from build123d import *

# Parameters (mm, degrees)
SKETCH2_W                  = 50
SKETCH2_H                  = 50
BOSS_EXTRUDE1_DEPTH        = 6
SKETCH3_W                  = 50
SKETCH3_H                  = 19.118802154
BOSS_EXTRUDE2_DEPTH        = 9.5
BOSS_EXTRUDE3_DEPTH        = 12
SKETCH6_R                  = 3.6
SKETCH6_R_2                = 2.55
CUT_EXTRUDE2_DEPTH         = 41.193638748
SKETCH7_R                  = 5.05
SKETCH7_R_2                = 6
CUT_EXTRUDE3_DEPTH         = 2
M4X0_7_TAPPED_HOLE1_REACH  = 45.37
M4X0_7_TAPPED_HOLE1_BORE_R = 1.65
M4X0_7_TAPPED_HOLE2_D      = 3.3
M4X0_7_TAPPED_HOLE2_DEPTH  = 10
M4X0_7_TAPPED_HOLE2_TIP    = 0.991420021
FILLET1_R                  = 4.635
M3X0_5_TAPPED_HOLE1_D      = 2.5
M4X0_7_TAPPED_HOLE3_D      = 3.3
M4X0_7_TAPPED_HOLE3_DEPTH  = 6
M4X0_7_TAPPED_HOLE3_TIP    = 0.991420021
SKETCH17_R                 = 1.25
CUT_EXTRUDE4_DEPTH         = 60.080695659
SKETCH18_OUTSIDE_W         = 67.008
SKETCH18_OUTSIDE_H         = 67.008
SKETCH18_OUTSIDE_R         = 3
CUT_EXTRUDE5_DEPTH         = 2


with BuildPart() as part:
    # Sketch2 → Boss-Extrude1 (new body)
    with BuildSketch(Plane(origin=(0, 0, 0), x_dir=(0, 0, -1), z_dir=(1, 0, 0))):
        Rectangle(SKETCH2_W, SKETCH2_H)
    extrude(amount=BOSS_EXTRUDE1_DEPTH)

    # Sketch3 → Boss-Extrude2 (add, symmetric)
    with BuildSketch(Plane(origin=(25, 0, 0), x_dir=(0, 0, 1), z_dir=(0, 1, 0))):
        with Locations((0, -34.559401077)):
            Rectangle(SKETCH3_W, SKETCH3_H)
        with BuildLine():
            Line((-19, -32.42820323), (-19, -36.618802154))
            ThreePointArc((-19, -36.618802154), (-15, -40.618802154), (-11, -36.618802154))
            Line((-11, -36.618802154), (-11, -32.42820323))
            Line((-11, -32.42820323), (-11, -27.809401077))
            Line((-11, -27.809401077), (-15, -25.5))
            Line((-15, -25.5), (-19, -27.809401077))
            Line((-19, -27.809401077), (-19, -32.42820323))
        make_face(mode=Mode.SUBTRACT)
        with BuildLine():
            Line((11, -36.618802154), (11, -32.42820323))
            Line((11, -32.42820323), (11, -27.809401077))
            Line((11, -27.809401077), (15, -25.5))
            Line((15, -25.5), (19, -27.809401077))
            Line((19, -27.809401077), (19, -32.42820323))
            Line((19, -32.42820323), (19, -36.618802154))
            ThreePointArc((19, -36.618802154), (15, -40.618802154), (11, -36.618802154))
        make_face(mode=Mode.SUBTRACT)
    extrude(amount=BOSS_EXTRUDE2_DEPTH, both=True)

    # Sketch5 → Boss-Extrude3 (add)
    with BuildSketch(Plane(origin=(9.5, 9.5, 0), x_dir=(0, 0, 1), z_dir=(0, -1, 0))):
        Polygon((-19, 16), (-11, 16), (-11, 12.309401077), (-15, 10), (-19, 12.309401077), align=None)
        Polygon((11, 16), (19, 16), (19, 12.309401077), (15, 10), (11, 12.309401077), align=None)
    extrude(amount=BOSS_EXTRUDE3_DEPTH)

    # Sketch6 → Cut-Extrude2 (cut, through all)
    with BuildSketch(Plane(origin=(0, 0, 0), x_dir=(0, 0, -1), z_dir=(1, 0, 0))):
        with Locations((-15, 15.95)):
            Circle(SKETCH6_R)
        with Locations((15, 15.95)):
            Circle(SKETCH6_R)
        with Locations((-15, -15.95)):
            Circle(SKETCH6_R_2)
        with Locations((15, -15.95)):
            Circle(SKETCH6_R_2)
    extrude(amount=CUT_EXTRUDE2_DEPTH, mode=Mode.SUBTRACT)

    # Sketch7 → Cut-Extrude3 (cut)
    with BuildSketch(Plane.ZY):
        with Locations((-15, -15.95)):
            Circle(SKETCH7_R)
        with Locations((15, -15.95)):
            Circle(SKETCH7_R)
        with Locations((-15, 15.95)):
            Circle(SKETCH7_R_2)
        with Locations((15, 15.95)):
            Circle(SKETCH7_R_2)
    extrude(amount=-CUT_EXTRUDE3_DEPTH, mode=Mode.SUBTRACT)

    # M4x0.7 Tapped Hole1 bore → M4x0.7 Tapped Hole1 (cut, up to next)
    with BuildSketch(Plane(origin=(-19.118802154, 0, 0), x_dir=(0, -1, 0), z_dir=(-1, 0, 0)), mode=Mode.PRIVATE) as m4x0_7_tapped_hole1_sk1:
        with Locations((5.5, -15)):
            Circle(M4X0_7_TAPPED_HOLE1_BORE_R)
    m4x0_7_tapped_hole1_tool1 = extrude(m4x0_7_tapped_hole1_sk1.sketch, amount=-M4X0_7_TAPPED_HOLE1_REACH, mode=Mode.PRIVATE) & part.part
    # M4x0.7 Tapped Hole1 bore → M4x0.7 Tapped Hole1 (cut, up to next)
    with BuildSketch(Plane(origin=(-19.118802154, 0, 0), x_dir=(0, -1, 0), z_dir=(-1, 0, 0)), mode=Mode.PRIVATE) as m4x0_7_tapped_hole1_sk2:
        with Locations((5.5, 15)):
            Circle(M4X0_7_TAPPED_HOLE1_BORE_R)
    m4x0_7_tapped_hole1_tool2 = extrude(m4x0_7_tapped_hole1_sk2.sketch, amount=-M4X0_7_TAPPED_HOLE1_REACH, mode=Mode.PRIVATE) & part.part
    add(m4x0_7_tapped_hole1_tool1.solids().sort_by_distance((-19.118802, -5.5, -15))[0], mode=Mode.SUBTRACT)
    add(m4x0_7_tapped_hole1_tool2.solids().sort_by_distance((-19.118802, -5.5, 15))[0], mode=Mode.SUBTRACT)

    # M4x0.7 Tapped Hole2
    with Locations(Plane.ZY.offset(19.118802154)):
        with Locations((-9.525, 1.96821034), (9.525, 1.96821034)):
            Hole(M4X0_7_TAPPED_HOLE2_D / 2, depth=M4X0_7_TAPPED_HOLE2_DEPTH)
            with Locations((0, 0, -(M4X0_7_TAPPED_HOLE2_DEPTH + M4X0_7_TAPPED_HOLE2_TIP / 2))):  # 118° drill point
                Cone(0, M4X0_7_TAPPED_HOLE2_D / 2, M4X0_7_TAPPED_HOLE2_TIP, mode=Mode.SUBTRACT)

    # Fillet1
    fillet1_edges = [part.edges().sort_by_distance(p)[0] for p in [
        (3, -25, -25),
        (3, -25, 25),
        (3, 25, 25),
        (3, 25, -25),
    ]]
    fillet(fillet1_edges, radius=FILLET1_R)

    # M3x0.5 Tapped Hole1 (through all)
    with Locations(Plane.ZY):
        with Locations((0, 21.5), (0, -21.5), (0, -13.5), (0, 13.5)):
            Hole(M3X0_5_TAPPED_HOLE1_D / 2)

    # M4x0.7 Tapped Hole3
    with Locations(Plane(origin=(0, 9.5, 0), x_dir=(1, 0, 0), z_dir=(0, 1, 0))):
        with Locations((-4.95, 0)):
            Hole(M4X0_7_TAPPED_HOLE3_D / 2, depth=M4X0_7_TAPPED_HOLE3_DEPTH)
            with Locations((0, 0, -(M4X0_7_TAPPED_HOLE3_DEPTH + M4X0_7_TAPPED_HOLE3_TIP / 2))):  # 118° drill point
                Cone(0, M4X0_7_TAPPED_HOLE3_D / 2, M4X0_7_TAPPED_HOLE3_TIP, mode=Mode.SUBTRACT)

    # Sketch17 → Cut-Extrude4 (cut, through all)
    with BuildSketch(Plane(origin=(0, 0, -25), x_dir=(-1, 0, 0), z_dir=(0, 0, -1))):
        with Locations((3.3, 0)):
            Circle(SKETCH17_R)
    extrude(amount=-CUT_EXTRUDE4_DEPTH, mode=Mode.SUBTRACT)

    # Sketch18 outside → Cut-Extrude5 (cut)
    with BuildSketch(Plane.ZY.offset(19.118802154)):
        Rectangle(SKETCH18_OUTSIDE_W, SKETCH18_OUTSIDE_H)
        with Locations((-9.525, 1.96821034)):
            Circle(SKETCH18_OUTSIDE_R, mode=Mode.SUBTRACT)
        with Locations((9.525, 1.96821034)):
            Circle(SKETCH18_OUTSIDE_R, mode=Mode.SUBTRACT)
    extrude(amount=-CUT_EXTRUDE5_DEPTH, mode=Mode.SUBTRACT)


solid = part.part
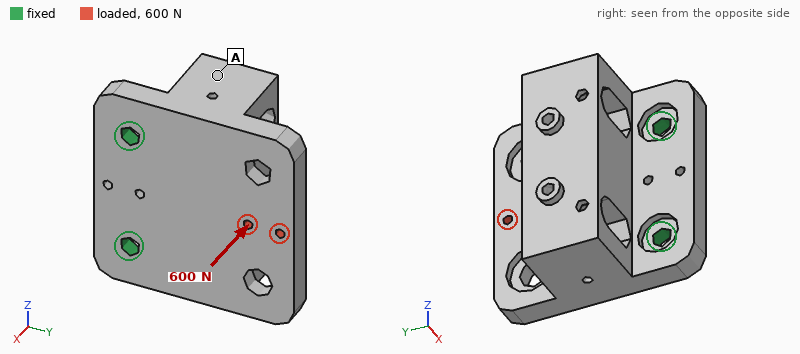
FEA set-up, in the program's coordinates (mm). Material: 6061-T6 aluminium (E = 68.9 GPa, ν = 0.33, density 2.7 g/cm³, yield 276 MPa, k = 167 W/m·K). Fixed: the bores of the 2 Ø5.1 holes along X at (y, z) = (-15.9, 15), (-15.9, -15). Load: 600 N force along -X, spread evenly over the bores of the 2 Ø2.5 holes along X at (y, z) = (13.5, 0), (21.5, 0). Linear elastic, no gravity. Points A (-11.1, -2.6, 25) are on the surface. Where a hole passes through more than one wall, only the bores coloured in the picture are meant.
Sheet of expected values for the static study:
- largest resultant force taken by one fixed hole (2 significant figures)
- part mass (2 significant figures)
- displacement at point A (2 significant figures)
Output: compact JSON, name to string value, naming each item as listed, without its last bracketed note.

{"largest resultant force taken by one fixed hole": "310 N", "part mass": "71 g", "displacement at point A": "0.077 mm"}
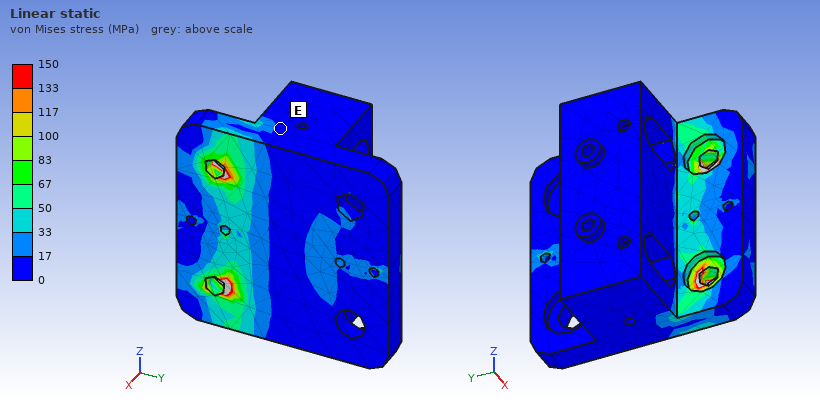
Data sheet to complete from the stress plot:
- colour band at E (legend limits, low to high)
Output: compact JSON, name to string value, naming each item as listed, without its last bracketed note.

{"colour band at E": "0 to 17 MPa"}
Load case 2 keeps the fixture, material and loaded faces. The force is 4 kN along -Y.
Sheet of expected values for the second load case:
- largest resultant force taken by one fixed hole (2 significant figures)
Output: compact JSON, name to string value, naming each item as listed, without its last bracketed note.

{"largest resultant force taken by one fixed hole": "2.0 kN"}
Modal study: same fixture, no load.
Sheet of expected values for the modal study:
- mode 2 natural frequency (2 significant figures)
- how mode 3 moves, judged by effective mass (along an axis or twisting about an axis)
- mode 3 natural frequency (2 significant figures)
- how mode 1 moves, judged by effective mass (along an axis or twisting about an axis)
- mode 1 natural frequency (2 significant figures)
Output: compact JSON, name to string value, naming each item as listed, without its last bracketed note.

{"mode 2 natural frequency": "6900 Hz", "how mode 3 moves, judged by effective mass": "along Z", "mode 3 natural frequency": "9700 Hz", "how mode 1 moves, judged by effective mass": "along X", "mode 1 natural frequency": "2000 Hz"}
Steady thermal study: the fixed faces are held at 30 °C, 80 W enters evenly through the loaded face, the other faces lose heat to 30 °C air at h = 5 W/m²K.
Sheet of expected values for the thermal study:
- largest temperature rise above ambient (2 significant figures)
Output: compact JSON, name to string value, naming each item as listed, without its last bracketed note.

{"largest temperature rise above ambient": "75 K"}
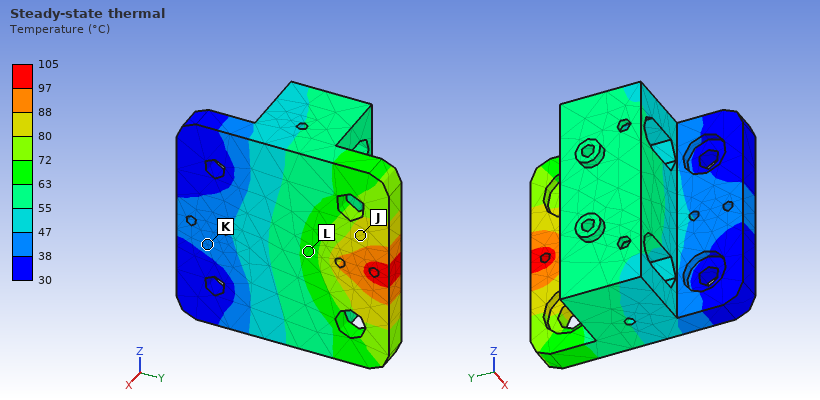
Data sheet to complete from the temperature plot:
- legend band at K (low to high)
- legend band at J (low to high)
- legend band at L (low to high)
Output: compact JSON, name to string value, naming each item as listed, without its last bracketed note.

{"legend band at K": "38 to 47 °C", "legend band at J": "80 to 88 °C", "legend band at L": "63 to 72 °C"}
